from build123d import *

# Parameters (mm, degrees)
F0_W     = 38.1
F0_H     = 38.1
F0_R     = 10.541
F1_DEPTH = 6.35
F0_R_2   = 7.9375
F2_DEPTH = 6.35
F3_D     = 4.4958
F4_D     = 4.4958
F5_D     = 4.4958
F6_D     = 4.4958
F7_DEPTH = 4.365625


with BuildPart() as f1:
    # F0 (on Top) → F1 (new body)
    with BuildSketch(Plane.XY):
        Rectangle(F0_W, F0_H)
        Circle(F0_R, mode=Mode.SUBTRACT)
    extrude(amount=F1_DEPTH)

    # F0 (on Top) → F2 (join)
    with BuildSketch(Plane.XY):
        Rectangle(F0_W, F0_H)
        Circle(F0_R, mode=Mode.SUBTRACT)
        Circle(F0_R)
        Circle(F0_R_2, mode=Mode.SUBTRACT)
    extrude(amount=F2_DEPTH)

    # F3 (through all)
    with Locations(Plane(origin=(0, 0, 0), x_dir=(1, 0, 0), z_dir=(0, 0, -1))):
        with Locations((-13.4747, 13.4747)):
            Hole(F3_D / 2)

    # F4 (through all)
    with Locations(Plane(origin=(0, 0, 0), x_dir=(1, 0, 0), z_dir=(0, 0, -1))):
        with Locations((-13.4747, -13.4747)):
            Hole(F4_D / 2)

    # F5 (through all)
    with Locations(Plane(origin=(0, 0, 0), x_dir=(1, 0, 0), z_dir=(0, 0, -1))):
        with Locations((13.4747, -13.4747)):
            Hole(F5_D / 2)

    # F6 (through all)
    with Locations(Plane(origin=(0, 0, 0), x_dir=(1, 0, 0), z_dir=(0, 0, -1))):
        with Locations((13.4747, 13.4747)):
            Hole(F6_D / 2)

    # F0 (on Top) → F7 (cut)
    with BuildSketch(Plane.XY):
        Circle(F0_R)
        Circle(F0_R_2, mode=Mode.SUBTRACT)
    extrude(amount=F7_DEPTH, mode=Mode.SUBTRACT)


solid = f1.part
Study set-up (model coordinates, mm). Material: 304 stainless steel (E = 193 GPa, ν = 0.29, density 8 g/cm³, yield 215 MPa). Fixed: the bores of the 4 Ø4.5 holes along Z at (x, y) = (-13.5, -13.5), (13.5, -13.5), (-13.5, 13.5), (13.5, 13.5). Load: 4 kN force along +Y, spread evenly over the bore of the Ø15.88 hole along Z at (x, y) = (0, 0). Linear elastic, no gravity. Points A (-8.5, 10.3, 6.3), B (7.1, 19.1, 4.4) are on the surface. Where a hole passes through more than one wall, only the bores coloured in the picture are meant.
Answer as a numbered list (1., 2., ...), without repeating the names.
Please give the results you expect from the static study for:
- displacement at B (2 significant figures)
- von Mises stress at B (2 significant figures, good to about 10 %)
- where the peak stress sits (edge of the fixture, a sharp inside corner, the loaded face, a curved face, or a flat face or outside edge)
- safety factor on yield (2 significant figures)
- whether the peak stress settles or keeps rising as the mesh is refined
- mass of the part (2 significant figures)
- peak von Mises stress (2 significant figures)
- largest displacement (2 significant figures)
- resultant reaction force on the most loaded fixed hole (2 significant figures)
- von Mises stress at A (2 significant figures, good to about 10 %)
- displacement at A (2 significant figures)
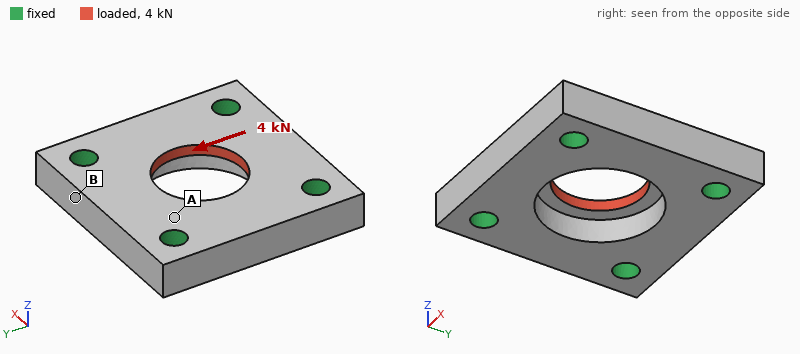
1. 1.2 µm
2. 11 MPa
3. the loaded face
4. 2.9
5. settles
6. 55 g
7. 73 MPa
8. 3.6 µm
9. 1.0 kN
10. 37 MPa
11. 0.98 µm
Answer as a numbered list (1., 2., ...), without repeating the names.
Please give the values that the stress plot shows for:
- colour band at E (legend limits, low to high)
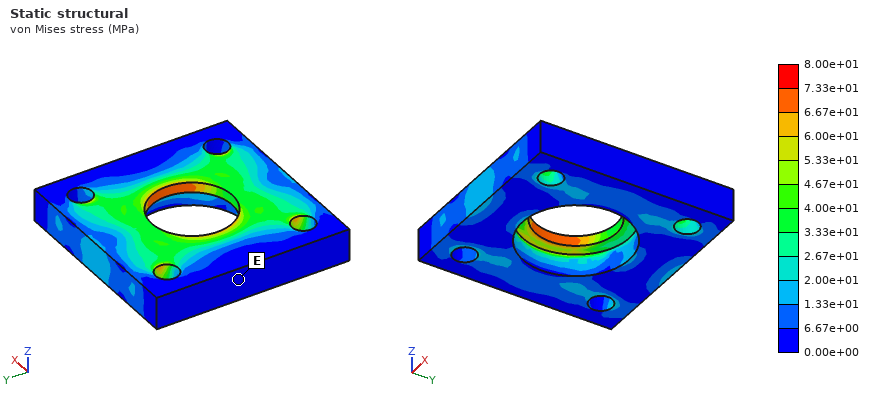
1. 0.00e+00 to 6.67e+00 MPa
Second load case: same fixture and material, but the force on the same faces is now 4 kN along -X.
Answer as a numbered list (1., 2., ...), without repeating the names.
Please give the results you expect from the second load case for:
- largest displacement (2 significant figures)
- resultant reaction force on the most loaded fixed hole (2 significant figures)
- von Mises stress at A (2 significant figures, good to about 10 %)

1. 3.6 µm
2. 1.0 kN
3. 30 MPa
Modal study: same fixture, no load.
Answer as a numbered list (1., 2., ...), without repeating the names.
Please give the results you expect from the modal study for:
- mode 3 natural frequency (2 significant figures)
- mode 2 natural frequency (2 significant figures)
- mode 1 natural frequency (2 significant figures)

1. 40 kHz
2. 39 kHz
3. 38 kHz
